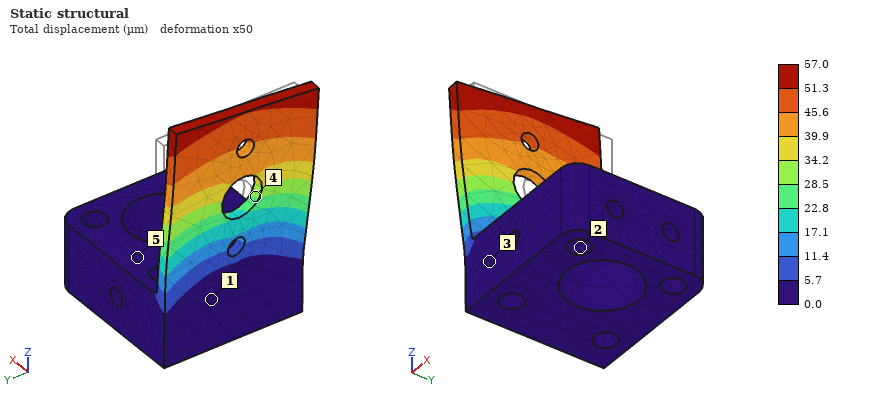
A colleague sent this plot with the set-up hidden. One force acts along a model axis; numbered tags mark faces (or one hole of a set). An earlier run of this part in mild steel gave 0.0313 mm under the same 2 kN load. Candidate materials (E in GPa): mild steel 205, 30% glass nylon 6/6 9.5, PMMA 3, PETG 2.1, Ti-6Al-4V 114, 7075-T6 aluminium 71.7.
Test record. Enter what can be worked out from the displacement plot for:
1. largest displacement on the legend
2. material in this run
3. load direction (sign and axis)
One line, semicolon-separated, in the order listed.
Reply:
57.0 µm; Ti-6Al-4V; -Y
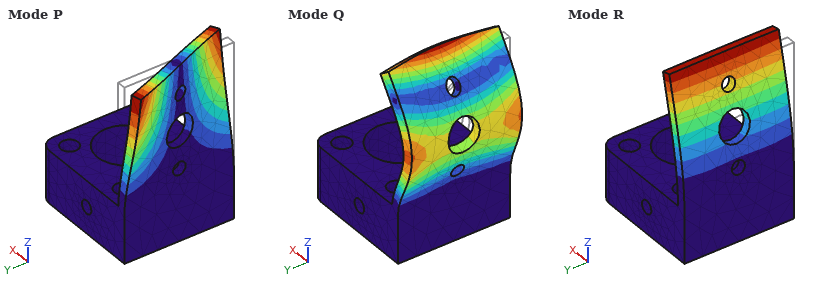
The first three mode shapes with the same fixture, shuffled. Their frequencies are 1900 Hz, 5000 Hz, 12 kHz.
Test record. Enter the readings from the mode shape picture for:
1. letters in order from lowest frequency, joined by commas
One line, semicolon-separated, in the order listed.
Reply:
R, P, Q
